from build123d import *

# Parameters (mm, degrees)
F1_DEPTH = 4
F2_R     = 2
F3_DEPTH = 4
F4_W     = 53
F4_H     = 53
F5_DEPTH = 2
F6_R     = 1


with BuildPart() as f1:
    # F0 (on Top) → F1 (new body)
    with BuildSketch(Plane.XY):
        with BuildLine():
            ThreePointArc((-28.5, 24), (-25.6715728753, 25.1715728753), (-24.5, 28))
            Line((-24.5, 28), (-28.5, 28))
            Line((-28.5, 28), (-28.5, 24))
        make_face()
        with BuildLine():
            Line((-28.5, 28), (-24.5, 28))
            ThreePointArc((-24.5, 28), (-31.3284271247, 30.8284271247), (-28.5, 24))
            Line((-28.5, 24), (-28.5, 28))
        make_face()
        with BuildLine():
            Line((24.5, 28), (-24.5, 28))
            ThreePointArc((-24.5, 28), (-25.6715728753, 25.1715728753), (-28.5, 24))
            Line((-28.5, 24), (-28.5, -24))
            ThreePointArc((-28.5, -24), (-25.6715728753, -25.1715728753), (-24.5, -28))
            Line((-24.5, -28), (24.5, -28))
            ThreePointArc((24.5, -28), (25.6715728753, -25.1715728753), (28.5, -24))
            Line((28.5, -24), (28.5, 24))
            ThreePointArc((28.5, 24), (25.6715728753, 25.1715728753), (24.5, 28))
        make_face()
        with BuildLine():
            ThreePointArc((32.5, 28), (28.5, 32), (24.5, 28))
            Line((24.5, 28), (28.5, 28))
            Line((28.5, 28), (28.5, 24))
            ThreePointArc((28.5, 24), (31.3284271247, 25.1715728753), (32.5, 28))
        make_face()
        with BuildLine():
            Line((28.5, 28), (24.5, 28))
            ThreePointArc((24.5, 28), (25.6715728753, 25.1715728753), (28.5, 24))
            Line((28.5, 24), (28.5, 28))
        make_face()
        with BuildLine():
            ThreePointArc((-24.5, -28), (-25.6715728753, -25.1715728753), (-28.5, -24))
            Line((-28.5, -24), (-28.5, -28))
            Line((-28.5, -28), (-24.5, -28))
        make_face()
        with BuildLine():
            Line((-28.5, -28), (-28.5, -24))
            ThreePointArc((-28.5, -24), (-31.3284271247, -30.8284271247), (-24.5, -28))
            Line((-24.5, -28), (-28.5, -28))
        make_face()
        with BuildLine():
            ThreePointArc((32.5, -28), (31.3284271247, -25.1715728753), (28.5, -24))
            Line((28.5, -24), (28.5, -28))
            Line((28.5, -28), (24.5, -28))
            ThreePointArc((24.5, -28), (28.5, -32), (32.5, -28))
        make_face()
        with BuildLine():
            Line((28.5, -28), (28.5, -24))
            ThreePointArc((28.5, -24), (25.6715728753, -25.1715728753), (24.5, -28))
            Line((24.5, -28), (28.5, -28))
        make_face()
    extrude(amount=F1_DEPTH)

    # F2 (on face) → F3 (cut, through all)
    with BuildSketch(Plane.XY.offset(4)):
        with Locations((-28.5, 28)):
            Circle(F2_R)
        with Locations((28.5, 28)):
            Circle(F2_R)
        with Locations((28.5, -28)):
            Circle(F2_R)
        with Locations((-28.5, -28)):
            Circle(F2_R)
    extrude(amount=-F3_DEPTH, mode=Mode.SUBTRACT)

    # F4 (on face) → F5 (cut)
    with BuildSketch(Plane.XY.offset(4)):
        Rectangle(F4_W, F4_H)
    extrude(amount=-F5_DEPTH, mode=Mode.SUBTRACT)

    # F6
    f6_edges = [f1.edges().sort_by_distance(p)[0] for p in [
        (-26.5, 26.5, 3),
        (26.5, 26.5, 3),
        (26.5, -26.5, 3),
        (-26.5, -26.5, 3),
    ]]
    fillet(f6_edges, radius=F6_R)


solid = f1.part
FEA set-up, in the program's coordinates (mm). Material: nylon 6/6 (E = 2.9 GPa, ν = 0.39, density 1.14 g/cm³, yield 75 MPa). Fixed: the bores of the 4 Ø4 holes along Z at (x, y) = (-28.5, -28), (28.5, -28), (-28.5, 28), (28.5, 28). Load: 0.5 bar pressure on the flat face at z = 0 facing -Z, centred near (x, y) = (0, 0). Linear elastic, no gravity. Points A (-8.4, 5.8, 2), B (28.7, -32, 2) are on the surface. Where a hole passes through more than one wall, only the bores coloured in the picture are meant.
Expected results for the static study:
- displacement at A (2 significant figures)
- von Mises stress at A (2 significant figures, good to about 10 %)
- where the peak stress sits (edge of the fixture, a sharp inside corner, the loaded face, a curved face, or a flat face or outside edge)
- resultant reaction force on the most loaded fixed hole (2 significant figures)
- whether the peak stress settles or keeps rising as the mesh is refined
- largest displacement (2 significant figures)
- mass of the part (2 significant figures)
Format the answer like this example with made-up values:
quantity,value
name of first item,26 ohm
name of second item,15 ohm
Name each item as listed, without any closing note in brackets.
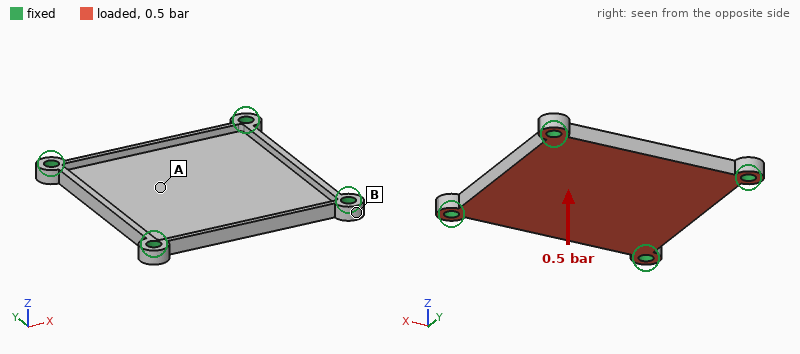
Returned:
quantity,value
displacement at A,0.91 mm
von Mises stress at A,9.3 MPa
where the peak stress sits,a sharp inside corner
resultant reaction force on the most loaded fixed hole,58 N
whether the peak stress settles or keeps rising as the mesh is refined,keeps rising
largest displacement,1.0 mm
mass of the part,8.6 g
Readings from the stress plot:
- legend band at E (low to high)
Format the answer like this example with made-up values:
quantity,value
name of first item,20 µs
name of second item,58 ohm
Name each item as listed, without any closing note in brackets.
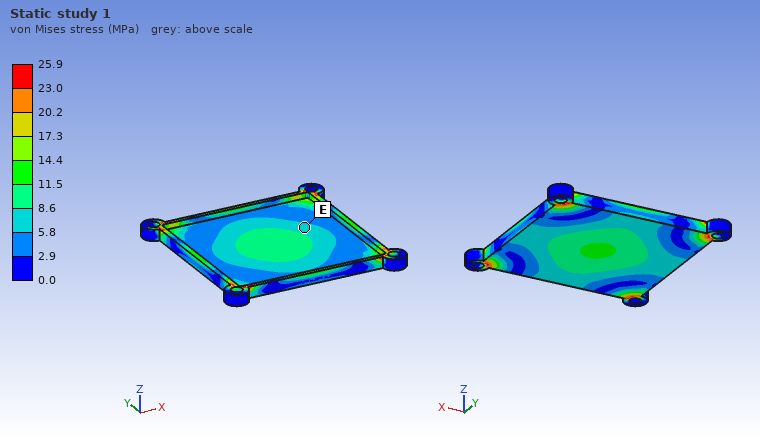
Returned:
quantity,value
legend band at E,5.8 to 8.6 MPa
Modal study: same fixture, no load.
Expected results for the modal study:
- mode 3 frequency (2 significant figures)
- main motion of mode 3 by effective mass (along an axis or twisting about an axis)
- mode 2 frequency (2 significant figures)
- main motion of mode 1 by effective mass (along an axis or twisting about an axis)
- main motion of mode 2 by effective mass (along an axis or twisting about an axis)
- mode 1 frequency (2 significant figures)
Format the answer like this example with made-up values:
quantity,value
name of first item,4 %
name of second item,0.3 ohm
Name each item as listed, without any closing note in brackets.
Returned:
quantity,value
mode 3 frequency,1700 Hz
main motion of mode 3 by effective mass,twisting about Y
mode 2 frequency,1700 Hz
main motion of mode 1 by effective mass,along Z
main motion of mode 2 by effective mass,twisting about X
mode 1 frequency,900 Hz
